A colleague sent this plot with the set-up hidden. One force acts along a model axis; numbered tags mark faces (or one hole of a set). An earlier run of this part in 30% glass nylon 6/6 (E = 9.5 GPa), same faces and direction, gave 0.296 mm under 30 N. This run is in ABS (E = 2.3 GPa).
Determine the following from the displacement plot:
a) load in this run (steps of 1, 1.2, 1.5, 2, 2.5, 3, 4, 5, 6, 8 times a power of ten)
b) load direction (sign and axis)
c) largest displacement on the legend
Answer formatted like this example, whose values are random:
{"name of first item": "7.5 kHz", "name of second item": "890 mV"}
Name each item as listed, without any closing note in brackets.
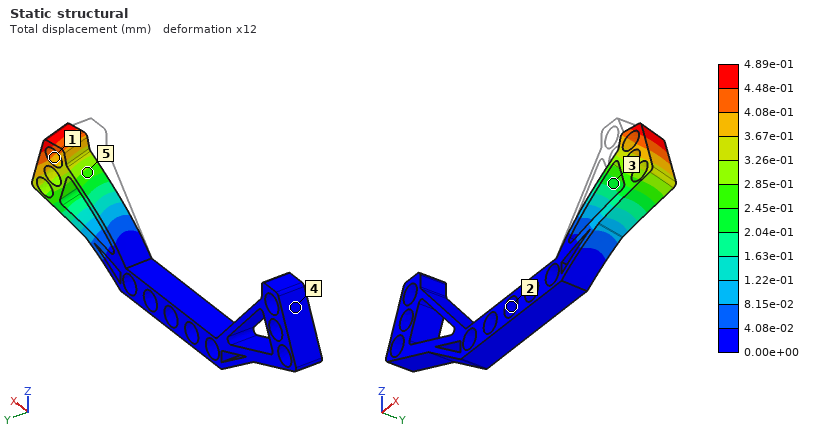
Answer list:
{"load in this run": "12 N", "load direction": "+Y", "largest displacement on the legend": "4.89e-01 mm"}
